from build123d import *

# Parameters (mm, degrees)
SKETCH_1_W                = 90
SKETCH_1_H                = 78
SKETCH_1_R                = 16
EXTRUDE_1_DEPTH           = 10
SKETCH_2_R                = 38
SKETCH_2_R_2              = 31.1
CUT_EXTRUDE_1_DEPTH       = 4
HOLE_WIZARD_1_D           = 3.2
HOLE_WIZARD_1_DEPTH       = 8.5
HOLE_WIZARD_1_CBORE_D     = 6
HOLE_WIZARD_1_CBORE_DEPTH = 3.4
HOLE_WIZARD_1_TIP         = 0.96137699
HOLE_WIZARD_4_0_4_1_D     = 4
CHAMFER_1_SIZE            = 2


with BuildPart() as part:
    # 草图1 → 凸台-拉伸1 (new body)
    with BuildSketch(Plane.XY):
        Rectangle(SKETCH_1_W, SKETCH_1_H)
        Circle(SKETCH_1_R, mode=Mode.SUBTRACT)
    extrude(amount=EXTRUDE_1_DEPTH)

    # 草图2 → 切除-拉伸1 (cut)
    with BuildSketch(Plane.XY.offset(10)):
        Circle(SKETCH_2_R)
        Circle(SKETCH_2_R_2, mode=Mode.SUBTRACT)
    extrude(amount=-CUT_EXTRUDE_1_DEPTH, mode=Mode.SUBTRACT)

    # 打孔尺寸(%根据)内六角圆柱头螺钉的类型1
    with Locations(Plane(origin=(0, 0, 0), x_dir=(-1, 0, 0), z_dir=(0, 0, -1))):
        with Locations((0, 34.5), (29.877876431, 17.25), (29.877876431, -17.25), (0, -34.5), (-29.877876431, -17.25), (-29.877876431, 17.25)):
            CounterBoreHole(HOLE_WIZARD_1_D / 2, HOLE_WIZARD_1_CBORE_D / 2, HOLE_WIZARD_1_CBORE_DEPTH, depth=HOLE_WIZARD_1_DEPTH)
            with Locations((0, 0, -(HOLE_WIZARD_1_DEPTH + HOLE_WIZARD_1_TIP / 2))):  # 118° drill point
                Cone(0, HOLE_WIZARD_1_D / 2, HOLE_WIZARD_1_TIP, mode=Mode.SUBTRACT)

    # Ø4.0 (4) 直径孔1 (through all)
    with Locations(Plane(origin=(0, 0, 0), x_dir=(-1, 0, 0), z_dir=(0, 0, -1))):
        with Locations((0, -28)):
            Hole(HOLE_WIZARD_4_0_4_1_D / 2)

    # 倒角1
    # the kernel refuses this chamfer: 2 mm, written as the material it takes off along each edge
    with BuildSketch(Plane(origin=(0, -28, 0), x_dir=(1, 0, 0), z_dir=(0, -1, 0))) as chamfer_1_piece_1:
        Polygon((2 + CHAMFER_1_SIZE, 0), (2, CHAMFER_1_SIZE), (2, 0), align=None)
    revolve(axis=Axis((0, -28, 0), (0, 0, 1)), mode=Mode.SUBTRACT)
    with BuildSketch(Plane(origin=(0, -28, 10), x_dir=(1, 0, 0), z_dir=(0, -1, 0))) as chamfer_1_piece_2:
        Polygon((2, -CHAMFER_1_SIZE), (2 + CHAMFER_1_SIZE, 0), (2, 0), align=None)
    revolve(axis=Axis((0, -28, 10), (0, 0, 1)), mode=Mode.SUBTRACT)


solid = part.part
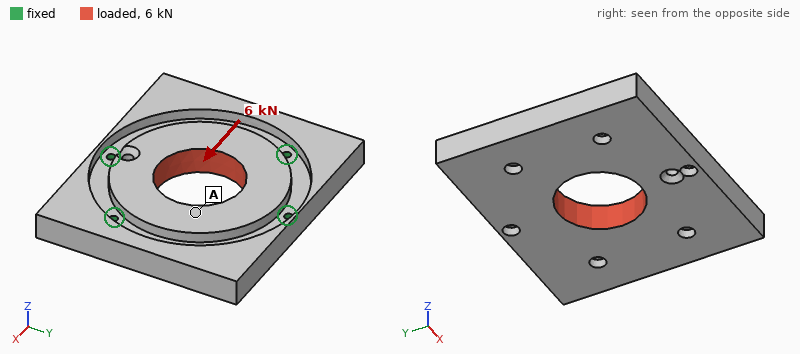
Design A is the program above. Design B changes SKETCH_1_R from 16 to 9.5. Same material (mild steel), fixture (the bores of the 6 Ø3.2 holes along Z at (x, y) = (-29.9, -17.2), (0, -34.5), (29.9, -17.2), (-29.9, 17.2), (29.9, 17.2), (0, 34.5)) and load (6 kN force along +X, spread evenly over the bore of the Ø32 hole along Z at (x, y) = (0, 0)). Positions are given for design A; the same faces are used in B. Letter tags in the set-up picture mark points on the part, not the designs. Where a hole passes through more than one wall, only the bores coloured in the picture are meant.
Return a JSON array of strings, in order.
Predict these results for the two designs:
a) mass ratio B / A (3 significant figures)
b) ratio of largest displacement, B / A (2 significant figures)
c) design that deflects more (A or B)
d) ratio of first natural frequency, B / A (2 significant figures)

["1.09", "1.2", "B", "1.0"]
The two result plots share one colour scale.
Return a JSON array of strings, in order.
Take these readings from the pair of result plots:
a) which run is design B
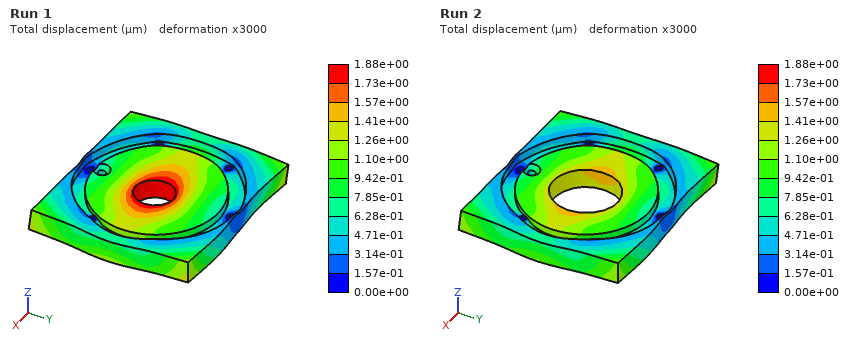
["Run 1"]
